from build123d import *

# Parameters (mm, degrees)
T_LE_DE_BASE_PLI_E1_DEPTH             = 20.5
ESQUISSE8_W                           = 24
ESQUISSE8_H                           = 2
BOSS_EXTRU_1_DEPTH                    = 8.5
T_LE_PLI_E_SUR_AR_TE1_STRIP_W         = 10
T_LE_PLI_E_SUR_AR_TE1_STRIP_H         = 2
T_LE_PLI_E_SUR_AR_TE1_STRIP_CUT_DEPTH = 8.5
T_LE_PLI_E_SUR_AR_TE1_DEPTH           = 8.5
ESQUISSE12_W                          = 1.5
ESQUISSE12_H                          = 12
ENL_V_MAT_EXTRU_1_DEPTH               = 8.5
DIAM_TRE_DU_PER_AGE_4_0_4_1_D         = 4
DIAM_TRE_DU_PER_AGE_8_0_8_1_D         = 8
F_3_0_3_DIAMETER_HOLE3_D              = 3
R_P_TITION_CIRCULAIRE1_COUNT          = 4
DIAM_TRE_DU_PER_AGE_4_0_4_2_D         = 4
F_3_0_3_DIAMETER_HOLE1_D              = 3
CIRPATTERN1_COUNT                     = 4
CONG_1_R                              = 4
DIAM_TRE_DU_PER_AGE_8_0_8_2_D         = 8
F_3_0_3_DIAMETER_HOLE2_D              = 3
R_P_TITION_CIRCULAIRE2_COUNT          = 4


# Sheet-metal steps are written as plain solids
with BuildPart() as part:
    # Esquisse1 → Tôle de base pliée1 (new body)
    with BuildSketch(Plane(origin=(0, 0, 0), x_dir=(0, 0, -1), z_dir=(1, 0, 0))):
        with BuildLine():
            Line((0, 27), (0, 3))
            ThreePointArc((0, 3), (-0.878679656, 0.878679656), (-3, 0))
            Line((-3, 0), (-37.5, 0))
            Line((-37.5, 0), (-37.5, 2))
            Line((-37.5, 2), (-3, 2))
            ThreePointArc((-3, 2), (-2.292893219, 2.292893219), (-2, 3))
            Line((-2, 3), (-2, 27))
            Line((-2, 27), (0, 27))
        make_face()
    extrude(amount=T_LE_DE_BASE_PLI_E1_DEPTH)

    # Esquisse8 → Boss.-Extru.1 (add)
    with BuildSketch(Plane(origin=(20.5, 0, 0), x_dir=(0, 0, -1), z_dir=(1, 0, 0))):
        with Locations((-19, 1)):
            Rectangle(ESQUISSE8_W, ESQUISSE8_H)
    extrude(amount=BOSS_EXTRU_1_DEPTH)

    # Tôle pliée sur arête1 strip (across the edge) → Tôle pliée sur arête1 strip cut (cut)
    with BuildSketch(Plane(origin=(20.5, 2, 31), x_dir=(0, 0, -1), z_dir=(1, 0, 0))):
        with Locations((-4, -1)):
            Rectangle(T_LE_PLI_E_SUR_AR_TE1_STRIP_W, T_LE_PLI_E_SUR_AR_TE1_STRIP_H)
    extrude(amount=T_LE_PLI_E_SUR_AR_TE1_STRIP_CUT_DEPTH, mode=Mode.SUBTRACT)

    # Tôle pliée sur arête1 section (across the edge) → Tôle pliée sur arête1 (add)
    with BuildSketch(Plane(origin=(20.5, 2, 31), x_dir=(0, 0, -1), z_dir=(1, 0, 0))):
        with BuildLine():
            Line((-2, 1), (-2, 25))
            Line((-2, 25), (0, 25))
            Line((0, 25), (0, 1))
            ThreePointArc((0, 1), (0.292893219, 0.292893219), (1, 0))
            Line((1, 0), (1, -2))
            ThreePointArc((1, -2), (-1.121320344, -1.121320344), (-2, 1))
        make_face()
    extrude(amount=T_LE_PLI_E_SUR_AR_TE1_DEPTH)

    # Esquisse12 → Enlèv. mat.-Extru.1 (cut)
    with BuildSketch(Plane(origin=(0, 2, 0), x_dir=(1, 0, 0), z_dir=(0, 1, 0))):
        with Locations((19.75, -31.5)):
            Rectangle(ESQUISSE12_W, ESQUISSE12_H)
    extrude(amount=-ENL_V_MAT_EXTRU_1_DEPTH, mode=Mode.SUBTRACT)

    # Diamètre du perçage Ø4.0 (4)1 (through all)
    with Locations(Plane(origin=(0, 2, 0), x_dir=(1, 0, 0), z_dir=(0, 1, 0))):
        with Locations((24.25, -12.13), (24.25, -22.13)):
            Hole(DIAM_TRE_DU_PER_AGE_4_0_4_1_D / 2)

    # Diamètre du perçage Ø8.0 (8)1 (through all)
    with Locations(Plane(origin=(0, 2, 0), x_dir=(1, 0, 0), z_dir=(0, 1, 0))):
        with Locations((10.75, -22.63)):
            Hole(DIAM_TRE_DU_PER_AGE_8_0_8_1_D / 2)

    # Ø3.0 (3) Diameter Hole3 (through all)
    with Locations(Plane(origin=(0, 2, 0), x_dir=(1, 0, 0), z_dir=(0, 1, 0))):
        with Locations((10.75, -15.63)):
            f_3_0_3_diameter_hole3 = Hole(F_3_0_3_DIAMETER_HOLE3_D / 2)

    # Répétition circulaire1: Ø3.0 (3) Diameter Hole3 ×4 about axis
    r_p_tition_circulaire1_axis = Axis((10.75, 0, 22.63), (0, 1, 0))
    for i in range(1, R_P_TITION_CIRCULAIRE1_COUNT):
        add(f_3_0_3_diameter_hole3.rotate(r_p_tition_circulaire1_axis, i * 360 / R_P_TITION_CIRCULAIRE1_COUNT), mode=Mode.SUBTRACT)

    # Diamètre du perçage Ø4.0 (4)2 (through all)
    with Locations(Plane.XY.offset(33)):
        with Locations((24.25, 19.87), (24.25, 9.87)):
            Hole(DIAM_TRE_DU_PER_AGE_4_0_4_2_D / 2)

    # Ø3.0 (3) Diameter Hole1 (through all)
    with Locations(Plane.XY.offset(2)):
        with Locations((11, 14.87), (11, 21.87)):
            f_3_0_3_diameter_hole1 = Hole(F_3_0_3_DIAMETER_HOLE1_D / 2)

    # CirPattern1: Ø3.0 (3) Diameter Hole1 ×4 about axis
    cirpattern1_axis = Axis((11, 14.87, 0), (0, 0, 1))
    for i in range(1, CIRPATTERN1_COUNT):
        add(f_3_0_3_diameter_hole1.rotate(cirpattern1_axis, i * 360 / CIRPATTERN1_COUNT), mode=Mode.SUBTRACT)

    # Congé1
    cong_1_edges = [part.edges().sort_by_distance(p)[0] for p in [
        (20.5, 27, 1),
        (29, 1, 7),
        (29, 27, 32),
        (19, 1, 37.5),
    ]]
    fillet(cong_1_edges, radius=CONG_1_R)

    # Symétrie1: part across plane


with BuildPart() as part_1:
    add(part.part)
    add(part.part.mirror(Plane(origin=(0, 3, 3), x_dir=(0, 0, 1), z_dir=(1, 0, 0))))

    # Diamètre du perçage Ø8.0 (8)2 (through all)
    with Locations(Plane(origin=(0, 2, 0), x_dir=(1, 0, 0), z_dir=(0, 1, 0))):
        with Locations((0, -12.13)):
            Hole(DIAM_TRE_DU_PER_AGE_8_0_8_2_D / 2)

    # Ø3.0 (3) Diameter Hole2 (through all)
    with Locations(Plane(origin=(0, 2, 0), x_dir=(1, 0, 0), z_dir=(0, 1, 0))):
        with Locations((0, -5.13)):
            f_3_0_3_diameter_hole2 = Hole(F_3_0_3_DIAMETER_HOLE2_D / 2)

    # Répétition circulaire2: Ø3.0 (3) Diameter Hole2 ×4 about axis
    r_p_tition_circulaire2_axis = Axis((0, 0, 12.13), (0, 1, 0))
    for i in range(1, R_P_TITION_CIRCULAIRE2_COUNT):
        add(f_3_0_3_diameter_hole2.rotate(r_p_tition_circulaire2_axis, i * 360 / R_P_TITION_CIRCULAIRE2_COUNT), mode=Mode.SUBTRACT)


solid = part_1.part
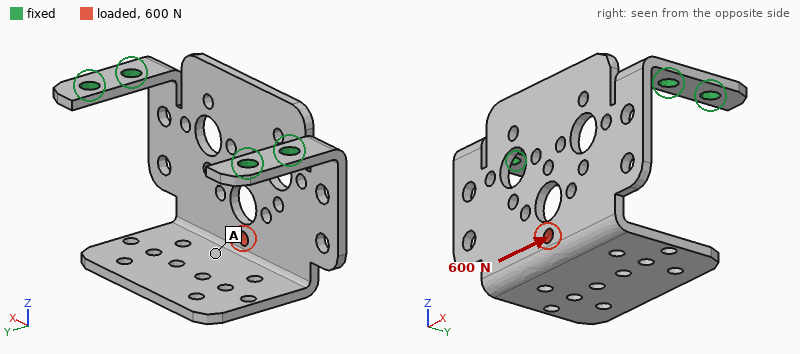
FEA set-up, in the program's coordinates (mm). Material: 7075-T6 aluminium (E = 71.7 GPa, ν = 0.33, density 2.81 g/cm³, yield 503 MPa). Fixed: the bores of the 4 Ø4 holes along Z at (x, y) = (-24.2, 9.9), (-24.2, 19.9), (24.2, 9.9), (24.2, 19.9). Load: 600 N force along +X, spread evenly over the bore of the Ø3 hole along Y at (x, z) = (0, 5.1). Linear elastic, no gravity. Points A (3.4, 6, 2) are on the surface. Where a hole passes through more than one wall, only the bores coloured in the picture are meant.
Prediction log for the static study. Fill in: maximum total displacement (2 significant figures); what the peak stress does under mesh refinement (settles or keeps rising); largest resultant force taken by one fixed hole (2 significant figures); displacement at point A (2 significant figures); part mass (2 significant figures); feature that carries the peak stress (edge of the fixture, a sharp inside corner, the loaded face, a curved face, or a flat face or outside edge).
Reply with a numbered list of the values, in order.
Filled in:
1. 0.37 mm
2. keeps rising
3. 470 N
4. 0.19 mm
5. 16 g
6. edge of the fixture
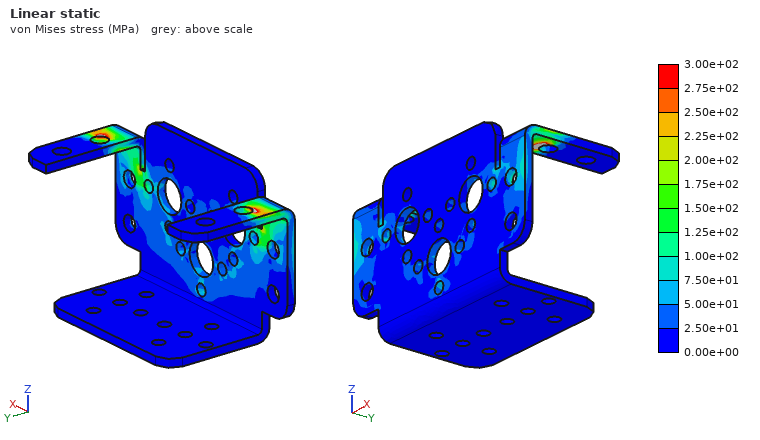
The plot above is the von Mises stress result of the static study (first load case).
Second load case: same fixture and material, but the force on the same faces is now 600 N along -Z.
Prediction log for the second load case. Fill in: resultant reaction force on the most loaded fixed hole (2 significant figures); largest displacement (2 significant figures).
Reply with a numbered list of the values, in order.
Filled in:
1. 310 N
2. 0.76 mm
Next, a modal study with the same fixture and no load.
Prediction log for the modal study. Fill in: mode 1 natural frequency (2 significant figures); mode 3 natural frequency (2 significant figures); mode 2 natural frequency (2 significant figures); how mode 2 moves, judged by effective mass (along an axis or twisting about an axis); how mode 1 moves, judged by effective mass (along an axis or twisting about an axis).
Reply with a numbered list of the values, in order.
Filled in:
1. 380 Hz
2. 1400 Hz
3. 1100 Hz
4. along X
5. along Y
